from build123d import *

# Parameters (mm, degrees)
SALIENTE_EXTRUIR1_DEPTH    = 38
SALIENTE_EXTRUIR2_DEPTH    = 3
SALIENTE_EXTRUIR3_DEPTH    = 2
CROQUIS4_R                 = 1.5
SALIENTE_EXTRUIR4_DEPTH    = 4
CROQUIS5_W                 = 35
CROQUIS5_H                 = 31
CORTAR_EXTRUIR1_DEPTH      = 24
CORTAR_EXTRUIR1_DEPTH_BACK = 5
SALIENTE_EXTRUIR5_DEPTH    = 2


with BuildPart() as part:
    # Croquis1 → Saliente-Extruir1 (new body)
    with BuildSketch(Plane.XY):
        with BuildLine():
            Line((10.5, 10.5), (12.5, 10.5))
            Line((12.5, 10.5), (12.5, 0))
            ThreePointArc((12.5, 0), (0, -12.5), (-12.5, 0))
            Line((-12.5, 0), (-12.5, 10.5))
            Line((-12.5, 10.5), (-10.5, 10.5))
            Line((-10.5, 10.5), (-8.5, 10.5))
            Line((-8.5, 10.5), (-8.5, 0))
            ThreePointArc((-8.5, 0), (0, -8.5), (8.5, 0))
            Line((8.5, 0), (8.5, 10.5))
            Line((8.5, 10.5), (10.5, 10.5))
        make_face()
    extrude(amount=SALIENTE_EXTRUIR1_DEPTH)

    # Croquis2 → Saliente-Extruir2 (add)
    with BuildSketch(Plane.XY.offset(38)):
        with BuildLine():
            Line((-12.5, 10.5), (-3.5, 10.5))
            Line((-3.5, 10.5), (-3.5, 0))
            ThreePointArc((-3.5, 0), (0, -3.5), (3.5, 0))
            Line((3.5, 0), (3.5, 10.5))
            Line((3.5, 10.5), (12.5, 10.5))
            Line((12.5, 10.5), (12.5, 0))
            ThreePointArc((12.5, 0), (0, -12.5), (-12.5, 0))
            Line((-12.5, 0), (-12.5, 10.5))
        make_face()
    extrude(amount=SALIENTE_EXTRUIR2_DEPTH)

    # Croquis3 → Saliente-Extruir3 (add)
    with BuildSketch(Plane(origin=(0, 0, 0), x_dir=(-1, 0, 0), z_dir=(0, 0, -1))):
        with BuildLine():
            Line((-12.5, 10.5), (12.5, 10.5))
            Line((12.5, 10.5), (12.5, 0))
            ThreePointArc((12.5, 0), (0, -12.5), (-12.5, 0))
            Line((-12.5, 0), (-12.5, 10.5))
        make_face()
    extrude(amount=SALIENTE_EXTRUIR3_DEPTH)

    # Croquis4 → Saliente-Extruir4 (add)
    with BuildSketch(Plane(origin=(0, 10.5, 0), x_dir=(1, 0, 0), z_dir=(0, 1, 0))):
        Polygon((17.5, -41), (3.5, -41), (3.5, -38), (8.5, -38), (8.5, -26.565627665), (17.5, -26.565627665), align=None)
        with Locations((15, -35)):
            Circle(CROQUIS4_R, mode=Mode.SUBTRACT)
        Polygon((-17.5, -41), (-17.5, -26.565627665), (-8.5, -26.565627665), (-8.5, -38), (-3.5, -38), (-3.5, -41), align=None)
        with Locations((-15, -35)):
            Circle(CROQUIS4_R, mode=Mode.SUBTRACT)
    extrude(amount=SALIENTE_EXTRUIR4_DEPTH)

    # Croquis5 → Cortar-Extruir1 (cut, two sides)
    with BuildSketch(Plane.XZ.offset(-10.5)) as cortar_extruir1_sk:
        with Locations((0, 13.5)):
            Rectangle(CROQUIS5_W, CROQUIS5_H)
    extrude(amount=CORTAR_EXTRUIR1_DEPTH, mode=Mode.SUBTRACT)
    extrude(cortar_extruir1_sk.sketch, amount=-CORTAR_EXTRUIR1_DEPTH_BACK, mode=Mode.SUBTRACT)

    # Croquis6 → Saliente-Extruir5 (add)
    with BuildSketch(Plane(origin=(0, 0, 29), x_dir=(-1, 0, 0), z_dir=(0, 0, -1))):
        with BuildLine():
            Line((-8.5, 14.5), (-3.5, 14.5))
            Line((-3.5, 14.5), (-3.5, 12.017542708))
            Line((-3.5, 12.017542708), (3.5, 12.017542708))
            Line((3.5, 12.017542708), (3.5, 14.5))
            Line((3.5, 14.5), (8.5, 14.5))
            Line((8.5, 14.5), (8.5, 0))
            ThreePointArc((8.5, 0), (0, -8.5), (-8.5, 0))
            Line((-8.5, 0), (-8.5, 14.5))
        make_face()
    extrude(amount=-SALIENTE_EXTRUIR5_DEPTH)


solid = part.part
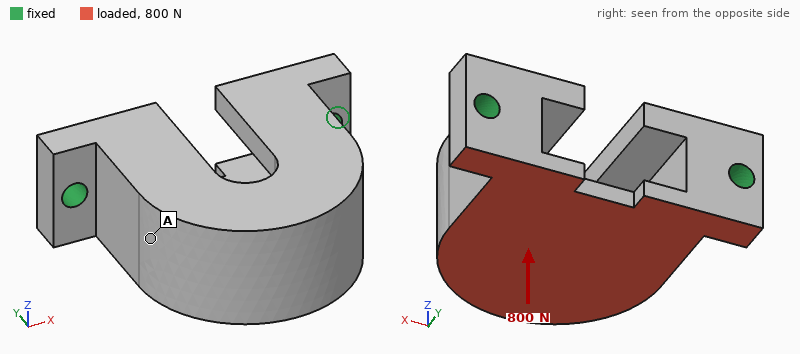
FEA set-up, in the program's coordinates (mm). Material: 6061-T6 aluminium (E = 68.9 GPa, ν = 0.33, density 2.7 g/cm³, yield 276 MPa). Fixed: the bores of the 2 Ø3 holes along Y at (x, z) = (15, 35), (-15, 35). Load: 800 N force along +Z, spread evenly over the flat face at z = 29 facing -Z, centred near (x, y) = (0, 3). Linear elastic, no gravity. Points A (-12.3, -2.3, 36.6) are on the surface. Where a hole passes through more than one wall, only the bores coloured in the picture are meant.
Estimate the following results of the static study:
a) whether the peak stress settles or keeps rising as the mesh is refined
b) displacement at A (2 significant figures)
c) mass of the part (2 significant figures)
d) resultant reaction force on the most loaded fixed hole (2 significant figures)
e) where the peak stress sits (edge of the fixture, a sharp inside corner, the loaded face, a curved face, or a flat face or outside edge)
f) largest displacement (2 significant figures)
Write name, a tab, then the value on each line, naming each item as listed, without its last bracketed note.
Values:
whether the peak stress settles or keeps rising as the mesh is refined	keeps rising
displacement at A	46 µm
mass of the part	13 g
resultant reaction force on the most loaded fixed hole	420 N
where the peak stress sits	edge of the fixture
largest displacement	80 µm
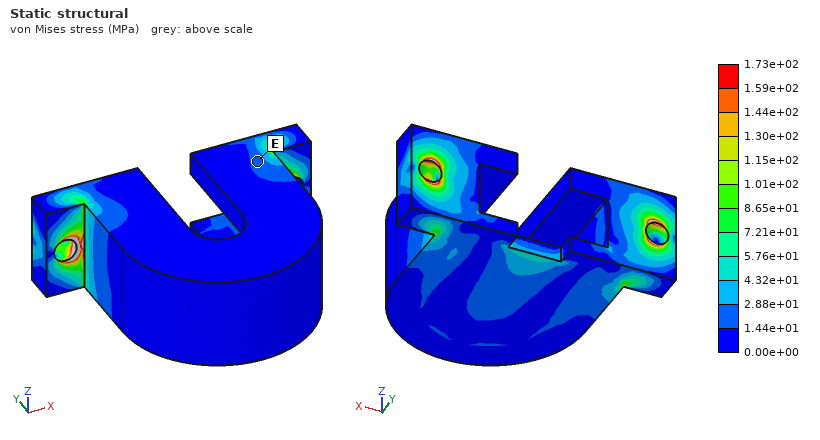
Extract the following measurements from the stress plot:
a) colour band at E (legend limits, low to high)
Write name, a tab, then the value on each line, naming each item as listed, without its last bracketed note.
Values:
colour band at E	1.44e+01 to 2.88e+01 MPa
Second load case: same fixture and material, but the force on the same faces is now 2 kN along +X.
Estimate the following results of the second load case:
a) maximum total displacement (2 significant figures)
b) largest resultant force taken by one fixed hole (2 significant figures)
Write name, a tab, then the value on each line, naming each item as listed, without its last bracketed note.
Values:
maximum total displacement	24 µm
largest resultant force taken by one fixed hole	1.3 kN
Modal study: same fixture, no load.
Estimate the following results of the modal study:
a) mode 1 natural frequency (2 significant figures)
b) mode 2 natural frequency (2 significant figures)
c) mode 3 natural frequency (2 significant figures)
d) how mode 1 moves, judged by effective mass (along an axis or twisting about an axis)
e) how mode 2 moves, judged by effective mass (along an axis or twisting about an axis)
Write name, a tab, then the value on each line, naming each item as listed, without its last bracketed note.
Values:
mode 1 natural frequency	5200 Hz
mode 2 natural frequency	14 kHz
mode 3 natural frequency	20 kHz
how mode 1 moves, judged by effective mass	along Z
how mode 2 moves, judged by effective mass	along X
